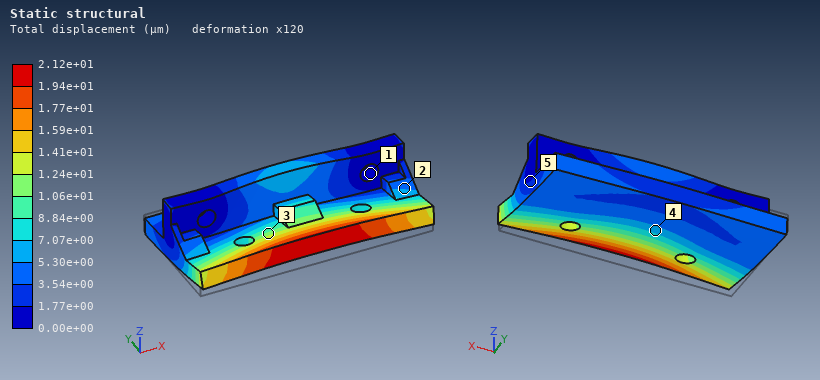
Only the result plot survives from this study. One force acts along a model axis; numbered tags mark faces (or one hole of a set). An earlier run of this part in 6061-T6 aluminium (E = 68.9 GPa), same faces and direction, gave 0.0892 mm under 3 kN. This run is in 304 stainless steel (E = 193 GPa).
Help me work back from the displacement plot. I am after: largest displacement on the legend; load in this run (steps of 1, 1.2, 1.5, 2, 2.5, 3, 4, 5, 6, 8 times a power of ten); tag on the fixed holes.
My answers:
2.12e+01 µm
2 kN
1
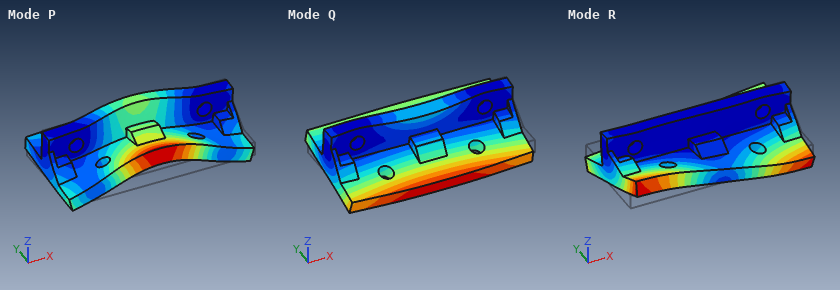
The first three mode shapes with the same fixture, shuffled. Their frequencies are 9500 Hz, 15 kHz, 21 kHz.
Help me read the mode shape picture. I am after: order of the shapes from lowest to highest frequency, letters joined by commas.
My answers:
Q, R, P
